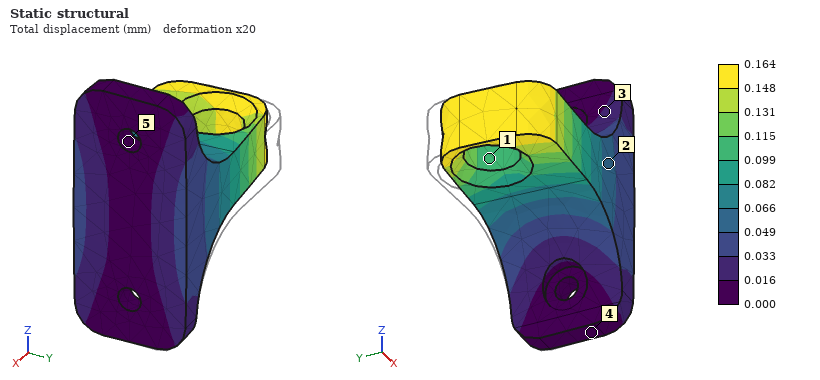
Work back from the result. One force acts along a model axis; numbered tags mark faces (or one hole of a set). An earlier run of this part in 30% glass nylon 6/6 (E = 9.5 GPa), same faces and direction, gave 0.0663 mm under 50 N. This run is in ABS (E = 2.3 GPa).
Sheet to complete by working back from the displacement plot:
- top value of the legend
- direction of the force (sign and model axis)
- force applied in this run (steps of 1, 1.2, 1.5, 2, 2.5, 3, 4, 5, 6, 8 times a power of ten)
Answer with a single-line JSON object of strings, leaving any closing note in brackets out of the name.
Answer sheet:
{"top value of the legend": "0.164 mm", "direction of the force": "-Y", "force applied in this run": "30 N"}
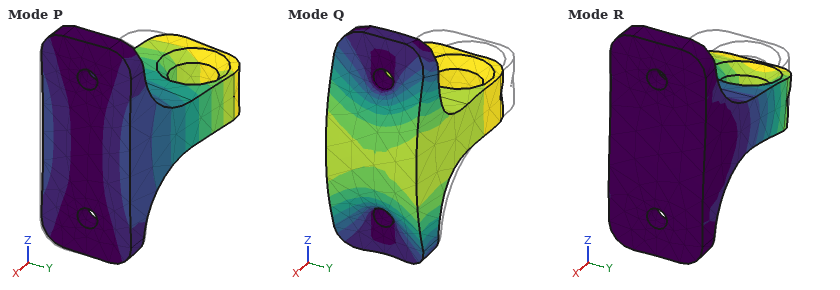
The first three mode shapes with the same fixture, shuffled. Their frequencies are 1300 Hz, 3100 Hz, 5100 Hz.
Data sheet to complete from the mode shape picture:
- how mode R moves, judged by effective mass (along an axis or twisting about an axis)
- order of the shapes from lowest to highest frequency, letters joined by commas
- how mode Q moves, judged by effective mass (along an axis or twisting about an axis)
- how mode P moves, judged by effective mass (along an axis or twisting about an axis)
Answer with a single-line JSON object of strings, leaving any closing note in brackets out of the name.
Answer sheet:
{"how mode R moves, judged by effective mass": "along Z", "order of the shapes from lowest to highest frequency, letters joined by commas": "P, R, Q", "how mode Q moves, judged by effective mass": "along X", "how mode P moves, judged by effective mass": "along Y"}
